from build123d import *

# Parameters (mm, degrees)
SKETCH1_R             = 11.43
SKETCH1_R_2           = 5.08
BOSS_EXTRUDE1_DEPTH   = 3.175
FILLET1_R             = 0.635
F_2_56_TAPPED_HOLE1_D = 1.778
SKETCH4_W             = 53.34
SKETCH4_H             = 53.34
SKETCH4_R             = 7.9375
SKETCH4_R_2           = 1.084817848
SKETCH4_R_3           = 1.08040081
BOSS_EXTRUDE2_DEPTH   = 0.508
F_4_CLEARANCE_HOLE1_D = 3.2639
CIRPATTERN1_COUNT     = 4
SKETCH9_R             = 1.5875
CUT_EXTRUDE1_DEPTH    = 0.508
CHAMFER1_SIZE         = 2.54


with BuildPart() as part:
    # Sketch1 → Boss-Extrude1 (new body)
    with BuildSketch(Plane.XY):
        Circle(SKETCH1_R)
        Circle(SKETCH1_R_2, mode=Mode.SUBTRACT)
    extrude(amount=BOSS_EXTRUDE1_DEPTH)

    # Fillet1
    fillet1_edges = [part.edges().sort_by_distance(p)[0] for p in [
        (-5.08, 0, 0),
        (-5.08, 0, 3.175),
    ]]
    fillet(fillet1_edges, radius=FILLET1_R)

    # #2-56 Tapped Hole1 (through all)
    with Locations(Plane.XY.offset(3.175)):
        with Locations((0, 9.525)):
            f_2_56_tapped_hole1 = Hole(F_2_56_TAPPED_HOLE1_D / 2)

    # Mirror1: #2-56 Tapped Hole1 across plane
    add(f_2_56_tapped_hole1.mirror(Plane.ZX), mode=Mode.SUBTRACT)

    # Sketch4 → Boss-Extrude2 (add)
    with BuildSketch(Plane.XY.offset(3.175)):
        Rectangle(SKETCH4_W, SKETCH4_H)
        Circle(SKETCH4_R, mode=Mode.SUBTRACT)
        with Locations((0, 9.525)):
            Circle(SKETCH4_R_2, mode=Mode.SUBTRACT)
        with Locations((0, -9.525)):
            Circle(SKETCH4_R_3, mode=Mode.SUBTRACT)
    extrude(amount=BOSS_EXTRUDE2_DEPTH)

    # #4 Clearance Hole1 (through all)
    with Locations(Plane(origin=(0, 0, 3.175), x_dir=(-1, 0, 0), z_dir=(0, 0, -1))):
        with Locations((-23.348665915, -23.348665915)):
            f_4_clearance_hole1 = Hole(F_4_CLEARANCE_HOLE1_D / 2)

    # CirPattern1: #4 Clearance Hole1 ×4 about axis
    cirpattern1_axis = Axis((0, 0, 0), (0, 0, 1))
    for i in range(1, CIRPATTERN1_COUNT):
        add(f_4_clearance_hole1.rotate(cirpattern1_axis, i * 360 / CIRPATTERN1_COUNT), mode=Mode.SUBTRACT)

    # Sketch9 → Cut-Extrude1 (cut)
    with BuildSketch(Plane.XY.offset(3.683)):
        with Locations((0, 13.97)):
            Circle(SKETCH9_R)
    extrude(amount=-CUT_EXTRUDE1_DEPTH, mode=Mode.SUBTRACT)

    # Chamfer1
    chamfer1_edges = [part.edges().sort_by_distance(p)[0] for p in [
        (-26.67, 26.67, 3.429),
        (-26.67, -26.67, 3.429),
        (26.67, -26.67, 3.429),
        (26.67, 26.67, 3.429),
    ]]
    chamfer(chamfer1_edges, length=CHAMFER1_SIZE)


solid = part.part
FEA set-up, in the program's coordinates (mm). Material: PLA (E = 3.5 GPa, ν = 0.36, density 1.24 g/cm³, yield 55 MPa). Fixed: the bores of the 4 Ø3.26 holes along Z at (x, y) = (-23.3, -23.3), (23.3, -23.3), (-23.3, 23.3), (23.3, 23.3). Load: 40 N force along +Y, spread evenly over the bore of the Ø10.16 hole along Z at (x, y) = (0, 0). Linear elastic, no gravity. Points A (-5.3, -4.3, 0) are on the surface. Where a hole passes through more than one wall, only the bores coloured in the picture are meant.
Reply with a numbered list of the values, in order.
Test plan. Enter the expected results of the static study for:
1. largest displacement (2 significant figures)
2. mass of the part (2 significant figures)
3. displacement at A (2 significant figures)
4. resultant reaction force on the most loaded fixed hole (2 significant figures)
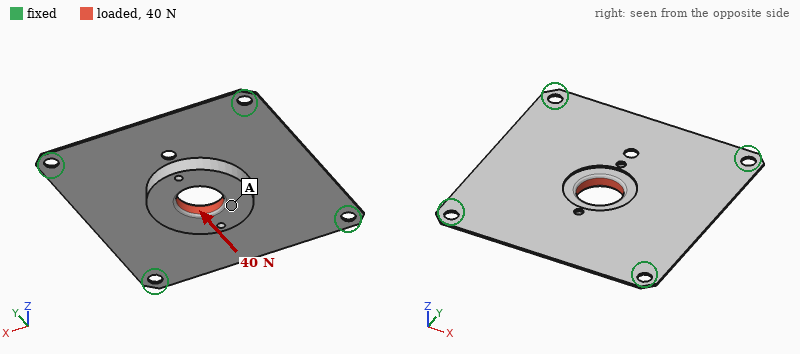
1. 0.79 mm
2. 2.9 g
3. 0.31 mm
4. 11 N
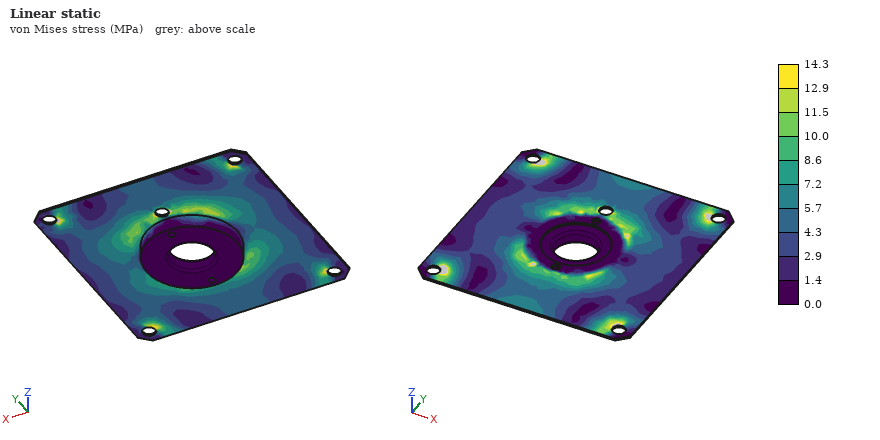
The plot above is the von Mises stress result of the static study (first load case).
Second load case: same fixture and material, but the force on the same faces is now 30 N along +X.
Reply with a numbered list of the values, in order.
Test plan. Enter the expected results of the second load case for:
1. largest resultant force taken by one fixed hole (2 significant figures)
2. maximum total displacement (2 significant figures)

1. 8.6 N
2. 0.60 mm
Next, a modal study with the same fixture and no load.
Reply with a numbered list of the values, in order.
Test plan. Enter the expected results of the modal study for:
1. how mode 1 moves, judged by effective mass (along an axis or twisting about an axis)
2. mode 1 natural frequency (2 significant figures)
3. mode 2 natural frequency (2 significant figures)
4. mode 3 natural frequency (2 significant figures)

1. along Z
2. 230 Hz
3. 450 Hz
4. 450 Hz
